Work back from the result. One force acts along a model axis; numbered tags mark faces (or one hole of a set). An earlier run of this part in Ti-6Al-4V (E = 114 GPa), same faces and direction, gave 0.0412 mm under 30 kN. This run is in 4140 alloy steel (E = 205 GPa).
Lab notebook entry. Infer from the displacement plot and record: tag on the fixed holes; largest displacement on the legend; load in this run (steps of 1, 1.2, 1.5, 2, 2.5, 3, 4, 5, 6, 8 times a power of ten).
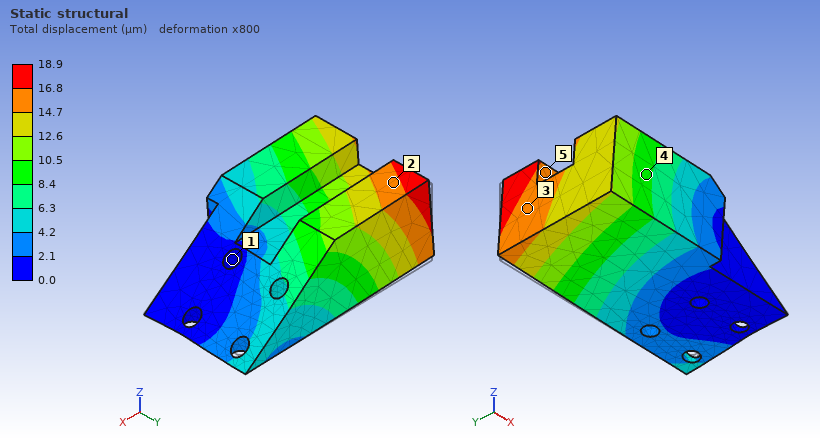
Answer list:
1
18.9 µm
25 kN
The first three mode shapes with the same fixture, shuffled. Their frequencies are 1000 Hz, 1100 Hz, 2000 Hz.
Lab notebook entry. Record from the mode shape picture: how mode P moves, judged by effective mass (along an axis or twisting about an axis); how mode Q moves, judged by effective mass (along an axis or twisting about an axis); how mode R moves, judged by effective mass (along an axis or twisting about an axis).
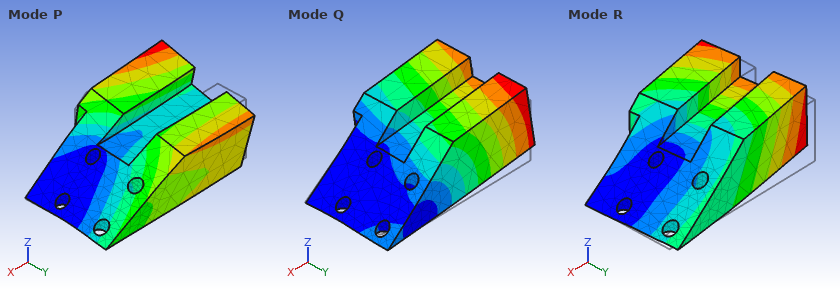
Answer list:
twisting about X
along Z
along Y
